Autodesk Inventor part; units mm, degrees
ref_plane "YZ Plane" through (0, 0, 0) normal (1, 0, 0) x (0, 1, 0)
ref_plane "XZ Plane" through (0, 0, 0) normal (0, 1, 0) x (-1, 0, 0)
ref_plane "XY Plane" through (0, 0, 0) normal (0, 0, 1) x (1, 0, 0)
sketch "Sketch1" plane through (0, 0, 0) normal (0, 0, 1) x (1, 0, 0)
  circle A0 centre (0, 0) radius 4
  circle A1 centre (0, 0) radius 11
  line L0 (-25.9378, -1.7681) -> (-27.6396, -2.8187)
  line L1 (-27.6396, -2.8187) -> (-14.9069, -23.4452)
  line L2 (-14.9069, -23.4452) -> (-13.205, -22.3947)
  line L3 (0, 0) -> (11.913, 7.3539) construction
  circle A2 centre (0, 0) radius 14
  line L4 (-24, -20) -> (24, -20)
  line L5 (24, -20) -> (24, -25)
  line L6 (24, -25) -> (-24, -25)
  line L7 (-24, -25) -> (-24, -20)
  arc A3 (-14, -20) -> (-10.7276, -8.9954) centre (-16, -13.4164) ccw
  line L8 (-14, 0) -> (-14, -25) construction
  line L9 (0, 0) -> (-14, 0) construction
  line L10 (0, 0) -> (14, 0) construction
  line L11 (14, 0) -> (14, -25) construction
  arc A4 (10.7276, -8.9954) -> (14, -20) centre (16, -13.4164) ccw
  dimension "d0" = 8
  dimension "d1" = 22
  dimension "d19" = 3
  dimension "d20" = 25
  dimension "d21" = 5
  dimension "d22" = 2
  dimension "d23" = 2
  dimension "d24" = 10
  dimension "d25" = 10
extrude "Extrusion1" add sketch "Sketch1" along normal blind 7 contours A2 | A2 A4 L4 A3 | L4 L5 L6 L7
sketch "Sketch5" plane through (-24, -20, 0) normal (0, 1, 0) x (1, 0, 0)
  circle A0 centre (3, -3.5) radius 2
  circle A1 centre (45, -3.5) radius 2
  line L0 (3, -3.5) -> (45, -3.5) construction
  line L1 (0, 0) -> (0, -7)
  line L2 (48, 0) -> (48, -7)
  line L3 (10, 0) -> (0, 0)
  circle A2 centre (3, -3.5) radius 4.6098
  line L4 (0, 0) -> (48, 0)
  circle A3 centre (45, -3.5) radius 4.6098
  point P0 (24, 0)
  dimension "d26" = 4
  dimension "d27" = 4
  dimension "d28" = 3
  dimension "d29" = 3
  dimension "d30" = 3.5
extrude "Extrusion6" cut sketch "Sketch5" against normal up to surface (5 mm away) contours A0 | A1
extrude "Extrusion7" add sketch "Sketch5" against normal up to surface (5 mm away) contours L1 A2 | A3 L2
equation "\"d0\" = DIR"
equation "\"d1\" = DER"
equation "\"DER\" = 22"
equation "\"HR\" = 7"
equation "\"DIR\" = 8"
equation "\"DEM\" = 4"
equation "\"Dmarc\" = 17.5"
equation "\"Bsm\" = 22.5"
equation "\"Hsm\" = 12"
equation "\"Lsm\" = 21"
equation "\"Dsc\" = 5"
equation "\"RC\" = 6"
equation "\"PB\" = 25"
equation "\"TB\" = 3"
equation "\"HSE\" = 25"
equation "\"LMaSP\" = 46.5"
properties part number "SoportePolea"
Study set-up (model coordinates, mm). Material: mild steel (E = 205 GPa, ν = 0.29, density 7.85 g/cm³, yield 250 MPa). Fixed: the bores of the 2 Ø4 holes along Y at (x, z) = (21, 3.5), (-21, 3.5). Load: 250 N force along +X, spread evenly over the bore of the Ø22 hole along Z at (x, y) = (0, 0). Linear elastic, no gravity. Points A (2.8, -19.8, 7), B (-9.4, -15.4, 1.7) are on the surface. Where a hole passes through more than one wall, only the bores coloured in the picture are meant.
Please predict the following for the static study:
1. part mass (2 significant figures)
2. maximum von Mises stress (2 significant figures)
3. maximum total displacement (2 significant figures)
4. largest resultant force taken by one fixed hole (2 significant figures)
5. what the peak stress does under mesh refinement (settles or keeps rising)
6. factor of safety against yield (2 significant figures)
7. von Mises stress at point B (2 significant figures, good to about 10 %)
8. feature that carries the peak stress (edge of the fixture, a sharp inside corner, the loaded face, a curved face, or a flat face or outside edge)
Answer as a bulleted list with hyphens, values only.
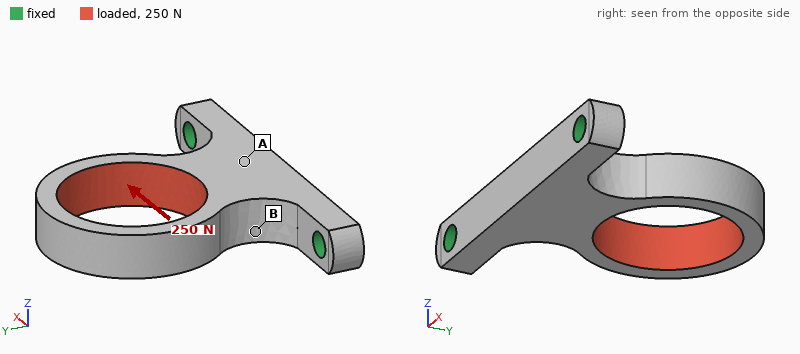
- 34 g
- 67 MPa
- 29 µm
- 220 N
- settles
- 3.7
- 23 MPa
- the loaded face
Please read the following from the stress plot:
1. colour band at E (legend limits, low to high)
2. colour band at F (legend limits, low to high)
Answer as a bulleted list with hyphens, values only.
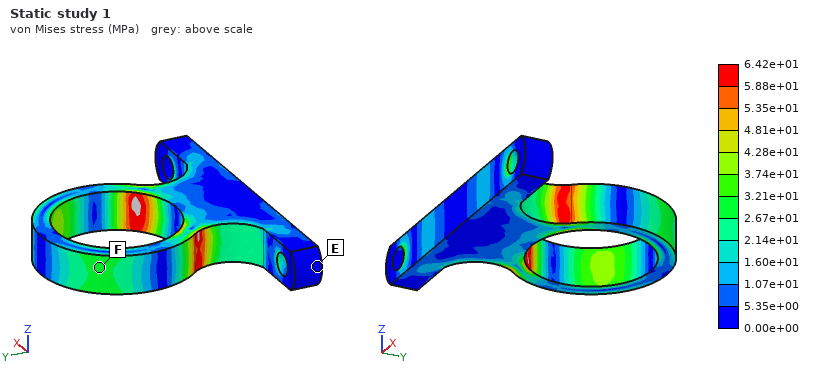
- 0.00e+00 to 5.35e+00 MPa
- 2.67e+01 to 3.21e+01 MPa
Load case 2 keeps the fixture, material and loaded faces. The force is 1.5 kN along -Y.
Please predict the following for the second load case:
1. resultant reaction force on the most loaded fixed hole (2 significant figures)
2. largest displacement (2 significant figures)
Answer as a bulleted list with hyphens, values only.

- 870 N
- 29 µm
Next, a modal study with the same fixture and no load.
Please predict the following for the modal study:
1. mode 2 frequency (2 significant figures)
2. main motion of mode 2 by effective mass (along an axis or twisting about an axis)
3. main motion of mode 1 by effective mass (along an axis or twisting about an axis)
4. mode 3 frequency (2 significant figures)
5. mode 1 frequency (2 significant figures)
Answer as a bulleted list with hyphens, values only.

- 4500 Hz
- along X
- along Z
- 9000 Hz
- 2500 Hz
